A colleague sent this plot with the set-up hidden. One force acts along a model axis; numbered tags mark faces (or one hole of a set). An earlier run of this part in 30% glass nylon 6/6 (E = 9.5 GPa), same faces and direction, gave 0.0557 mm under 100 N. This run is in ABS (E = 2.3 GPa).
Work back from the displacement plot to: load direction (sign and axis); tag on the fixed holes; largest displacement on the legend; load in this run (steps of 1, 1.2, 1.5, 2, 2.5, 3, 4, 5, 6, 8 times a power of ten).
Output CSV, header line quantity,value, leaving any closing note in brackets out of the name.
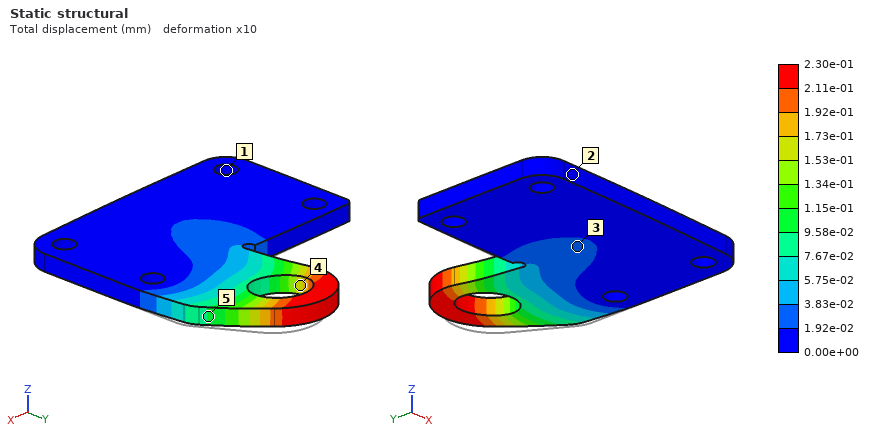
quantity,value
load direction,-X
tag on the fixed holes,1
largest displacement on the legend,2.30e-01 mm
load in this run,100 N
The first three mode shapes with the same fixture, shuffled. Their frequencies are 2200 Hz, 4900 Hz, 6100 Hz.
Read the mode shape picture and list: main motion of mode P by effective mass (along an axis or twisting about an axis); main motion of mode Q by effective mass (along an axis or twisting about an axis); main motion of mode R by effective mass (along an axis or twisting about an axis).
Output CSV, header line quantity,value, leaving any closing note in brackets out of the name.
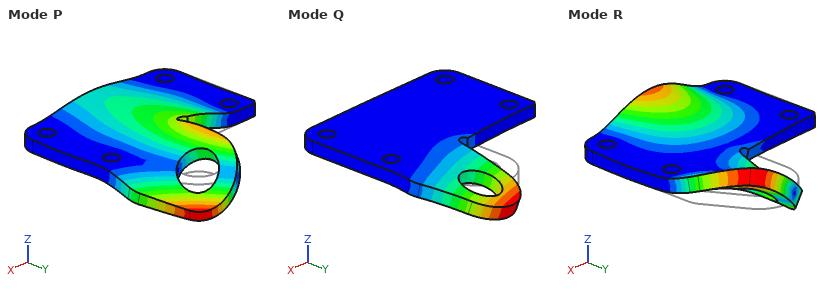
quantity,value
main motion of mode P by effective mass,along Z
main motion of mode Q by effective mass,along Z
main motion of mode R by effective mass,along Z
